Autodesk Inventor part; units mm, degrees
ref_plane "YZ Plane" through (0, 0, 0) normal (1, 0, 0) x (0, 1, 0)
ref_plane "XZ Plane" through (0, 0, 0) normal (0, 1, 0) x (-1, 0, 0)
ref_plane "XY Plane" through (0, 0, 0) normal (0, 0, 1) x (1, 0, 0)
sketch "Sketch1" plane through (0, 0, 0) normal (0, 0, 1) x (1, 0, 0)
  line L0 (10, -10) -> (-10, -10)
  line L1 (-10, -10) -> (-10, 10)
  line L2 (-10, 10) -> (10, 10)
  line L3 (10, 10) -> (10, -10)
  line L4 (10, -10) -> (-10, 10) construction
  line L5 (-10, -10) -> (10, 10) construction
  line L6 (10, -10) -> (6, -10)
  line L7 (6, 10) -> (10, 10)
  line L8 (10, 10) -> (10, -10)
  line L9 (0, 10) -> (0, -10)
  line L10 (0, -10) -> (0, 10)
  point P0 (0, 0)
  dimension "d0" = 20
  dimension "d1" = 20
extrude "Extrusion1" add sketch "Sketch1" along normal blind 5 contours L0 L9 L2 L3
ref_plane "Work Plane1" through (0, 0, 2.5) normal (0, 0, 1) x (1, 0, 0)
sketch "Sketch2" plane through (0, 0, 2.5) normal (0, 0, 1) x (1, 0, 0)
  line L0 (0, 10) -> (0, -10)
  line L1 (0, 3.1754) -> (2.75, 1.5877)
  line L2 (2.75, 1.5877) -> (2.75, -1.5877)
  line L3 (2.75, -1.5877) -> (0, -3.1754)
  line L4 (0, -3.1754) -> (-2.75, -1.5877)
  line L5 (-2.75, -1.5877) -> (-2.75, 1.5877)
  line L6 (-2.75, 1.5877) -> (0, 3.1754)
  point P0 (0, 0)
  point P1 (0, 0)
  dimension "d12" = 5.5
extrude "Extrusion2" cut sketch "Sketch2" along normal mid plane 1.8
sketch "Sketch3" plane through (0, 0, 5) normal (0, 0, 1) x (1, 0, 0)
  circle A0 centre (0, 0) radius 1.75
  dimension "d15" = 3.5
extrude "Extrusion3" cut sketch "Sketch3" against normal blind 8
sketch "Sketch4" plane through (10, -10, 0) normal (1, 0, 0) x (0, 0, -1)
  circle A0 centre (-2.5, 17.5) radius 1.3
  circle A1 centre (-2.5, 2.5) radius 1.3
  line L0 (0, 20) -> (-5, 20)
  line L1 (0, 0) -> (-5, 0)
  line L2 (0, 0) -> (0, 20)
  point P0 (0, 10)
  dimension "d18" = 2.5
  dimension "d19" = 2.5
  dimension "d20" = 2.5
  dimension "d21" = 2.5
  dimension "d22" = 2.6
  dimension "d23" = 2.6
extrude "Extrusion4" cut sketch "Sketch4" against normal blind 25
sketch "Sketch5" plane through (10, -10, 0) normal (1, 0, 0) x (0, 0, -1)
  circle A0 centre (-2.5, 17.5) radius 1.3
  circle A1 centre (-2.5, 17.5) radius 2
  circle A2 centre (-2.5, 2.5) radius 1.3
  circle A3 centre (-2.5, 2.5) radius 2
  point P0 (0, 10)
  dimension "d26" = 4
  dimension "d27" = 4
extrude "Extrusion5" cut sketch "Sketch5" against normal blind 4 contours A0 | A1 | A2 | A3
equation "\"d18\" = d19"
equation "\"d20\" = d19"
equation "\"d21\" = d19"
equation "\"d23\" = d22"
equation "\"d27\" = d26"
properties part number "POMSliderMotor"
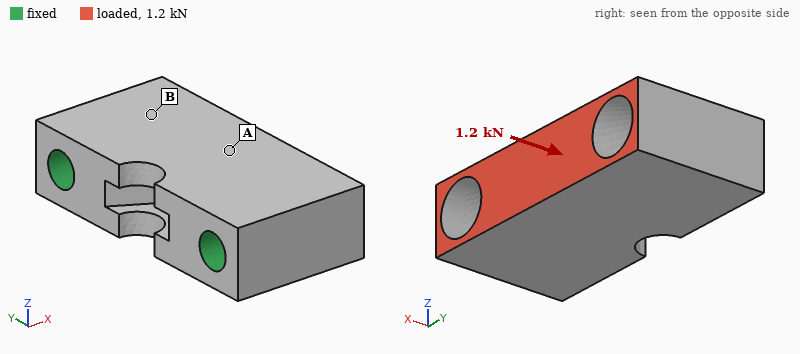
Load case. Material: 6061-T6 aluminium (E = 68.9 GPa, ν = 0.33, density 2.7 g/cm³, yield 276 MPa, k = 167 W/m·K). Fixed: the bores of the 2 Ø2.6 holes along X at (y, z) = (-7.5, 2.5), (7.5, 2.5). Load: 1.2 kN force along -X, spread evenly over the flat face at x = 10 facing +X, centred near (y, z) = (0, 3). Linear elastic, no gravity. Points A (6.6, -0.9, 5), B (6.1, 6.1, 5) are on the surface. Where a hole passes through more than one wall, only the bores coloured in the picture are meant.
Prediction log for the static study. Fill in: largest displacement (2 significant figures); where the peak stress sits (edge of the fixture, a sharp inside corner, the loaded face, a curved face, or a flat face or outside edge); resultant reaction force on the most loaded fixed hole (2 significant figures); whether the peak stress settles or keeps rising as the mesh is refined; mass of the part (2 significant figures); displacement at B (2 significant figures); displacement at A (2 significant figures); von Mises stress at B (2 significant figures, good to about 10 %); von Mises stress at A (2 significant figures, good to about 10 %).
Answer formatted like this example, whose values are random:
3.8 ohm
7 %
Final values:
3.3 µm
edge of the fixture
640 N
keeps rising
2.2 g
1.3 µm
2.8 µm
20 MPa
10 MPa
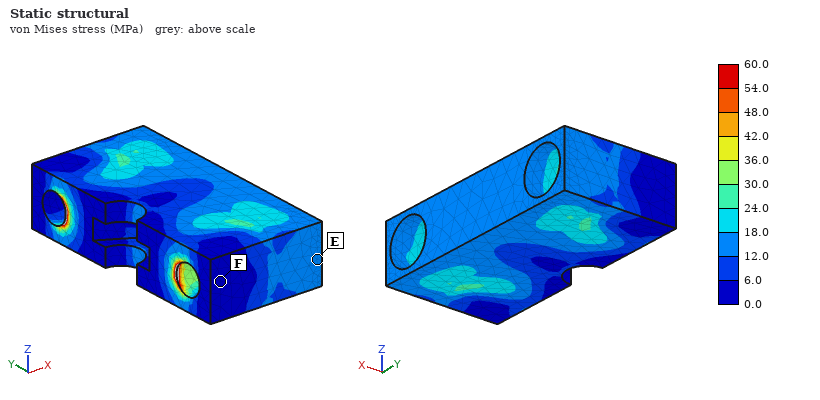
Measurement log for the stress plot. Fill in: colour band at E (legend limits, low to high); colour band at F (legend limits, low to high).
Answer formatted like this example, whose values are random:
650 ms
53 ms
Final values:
12.0 to 18.0 MPa
0.0 to 6.0 MPa
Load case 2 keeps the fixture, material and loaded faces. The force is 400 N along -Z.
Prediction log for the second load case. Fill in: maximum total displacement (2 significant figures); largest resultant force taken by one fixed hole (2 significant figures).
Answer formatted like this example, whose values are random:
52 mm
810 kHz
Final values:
9.6 µm
200 N
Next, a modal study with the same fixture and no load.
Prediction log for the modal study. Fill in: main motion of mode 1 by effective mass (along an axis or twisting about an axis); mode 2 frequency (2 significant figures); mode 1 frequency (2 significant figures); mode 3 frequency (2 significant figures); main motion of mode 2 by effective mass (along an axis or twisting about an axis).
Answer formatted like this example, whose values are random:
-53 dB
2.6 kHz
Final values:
along Z
87 kHz
50 kHz
91 kHz
along X
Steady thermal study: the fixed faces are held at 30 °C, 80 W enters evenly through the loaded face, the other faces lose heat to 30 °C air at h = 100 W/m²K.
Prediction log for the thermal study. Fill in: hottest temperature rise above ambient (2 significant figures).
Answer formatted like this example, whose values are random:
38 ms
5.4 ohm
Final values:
50 K
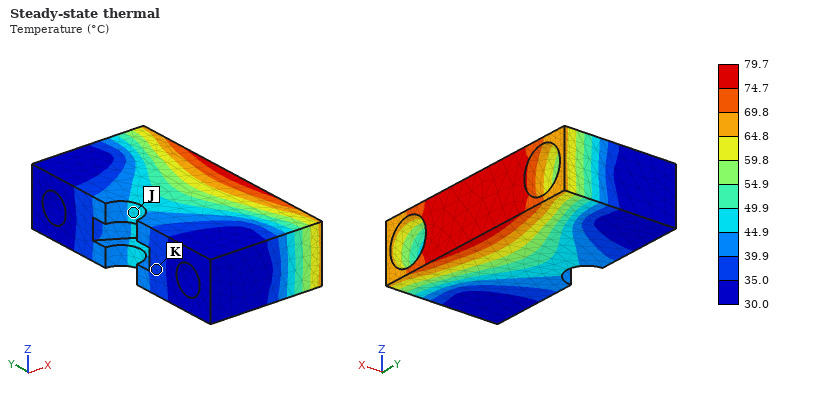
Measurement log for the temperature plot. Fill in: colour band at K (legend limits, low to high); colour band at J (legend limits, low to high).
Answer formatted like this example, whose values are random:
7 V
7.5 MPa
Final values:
35.0 to 39.9 °C
44.9 to 49.9 °C
